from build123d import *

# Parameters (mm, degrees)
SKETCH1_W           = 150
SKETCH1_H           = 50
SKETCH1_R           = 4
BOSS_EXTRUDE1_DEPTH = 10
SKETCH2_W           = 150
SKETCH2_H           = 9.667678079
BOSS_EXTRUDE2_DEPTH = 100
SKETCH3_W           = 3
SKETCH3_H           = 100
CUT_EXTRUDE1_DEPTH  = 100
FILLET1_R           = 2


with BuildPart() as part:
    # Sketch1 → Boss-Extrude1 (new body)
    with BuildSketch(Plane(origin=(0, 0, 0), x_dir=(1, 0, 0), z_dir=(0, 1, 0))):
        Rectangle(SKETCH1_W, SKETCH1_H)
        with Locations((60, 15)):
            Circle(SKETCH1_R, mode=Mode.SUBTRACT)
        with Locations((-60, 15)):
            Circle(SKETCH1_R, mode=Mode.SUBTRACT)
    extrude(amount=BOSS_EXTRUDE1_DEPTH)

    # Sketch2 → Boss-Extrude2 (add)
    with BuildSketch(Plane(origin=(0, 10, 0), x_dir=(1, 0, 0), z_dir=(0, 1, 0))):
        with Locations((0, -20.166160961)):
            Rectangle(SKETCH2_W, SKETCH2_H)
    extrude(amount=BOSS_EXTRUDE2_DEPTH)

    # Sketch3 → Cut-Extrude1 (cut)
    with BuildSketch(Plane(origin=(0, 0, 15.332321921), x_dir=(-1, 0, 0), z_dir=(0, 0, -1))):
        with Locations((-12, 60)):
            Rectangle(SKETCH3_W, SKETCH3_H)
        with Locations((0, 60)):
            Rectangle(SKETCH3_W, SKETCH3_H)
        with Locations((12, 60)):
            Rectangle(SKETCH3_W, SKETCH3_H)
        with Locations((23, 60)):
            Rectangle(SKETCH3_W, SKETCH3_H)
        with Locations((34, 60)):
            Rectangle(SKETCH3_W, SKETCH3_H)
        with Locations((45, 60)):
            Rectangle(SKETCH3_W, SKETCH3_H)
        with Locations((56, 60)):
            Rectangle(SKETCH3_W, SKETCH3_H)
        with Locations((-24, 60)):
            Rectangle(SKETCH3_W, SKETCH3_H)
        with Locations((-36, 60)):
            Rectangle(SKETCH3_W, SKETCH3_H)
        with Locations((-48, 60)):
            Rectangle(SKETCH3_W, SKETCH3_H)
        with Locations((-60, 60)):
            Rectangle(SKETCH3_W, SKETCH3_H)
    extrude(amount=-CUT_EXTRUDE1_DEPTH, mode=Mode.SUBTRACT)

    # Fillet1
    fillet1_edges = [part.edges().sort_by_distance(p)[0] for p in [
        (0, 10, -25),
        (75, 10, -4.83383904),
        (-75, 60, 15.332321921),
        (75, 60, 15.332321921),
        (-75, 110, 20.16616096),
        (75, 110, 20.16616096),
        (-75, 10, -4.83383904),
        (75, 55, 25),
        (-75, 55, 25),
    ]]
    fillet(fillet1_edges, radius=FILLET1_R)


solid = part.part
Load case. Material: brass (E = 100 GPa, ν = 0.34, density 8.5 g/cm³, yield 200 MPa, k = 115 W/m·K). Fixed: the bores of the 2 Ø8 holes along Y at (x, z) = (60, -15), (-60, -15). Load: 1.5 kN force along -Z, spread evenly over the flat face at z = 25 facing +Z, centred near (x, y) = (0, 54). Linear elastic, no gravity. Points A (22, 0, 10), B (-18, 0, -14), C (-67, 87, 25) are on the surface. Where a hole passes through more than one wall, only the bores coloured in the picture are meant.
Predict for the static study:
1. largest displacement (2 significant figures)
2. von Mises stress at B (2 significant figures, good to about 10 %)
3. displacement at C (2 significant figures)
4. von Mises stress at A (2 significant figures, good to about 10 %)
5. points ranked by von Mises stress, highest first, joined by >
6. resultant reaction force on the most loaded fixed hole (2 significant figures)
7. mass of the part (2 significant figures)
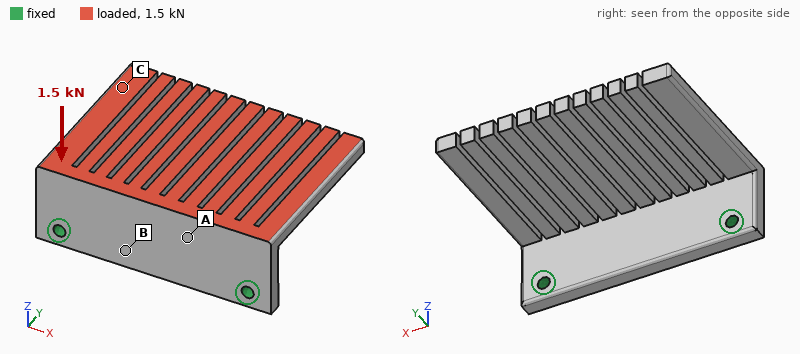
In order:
0.58 mm
13 MPa
0.38 mm
22 MPa
A > B > C
830 N
1.6 kg
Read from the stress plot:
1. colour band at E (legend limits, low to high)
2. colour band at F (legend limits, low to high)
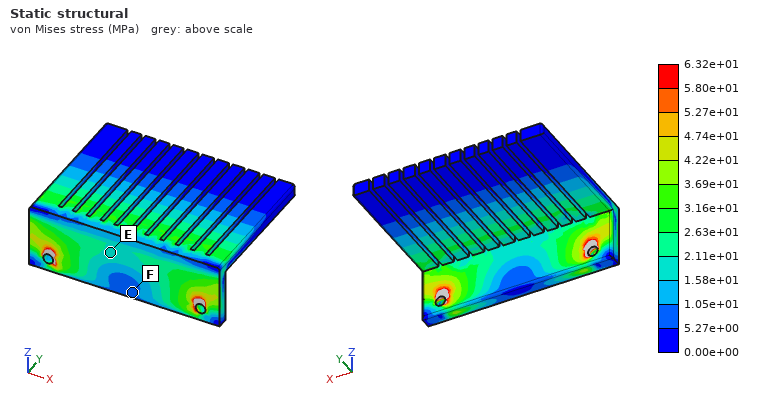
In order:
1.58e+01 to 2.11e+01 MPa
5.27e+00 to 1.05e+01 MPa
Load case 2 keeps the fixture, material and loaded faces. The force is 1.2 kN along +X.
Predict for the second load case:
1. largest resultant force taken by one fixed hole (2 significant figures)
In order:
830 N
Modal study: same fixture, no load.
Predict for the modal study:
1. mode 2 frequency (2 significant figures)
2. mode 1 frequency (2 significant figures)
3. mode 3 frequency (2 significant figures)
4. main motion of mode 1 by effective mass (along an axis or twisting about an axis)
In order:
360 Hz
300 Hz
370 Hz
along Z
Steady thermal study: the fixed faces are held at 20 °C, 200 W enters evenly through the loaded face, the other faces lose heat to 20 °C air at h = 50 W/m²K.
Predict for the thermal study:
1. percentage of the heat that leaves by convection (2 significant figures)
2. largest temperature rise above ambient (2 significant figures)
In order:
55 %
64 K
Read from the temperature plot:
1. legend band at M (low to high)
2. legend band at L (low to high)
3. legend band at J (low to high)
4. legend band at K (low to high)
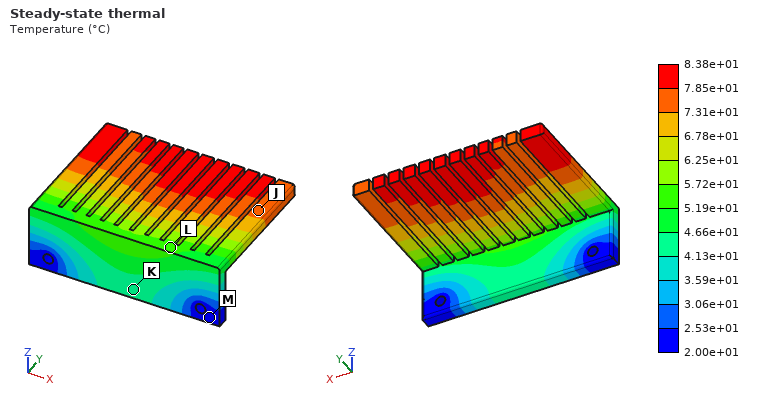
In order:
2.00e+01 to 2.53e+01 °C
5.19e+01 to 5.72e+01 °C
7.31e+01 to 7.85e+01 °C
4.13e+01 to 4.66e+01 °C
